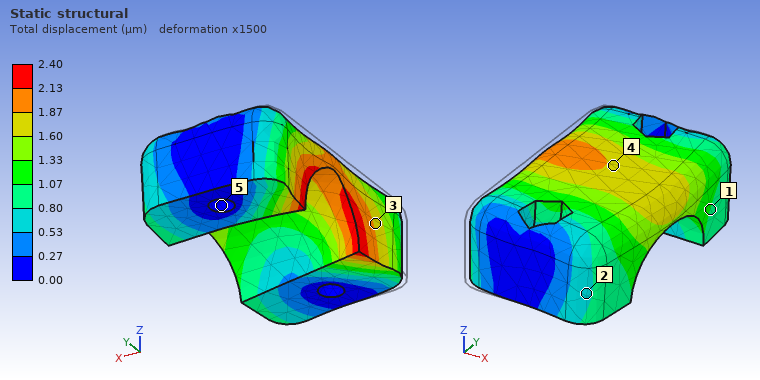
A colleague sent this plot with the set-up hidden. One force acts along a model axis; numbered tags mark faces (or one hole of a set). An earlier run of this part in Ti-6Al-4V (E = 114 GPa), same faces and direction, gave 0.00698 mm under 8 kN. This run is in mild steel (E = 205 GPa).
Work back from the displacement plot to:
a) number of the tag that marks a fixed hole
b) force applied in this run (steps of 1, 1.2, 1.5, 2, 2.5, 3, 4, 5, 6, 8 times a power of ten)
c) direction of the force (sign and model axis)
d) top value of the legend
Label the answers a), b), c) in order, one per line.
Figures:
a) 5
b) 5 kN
c) +X
d) 2.40 µm
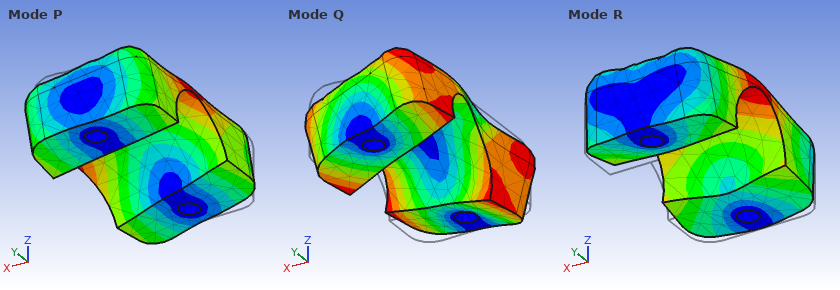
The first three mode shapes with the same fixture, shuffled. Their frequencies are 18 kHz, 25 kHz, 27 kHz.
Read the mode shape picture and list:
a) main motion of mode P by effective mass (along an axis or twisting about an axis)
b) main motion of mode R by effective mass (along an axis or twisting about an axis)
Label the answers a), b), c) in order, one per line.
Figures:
a) along X
b) along Z
